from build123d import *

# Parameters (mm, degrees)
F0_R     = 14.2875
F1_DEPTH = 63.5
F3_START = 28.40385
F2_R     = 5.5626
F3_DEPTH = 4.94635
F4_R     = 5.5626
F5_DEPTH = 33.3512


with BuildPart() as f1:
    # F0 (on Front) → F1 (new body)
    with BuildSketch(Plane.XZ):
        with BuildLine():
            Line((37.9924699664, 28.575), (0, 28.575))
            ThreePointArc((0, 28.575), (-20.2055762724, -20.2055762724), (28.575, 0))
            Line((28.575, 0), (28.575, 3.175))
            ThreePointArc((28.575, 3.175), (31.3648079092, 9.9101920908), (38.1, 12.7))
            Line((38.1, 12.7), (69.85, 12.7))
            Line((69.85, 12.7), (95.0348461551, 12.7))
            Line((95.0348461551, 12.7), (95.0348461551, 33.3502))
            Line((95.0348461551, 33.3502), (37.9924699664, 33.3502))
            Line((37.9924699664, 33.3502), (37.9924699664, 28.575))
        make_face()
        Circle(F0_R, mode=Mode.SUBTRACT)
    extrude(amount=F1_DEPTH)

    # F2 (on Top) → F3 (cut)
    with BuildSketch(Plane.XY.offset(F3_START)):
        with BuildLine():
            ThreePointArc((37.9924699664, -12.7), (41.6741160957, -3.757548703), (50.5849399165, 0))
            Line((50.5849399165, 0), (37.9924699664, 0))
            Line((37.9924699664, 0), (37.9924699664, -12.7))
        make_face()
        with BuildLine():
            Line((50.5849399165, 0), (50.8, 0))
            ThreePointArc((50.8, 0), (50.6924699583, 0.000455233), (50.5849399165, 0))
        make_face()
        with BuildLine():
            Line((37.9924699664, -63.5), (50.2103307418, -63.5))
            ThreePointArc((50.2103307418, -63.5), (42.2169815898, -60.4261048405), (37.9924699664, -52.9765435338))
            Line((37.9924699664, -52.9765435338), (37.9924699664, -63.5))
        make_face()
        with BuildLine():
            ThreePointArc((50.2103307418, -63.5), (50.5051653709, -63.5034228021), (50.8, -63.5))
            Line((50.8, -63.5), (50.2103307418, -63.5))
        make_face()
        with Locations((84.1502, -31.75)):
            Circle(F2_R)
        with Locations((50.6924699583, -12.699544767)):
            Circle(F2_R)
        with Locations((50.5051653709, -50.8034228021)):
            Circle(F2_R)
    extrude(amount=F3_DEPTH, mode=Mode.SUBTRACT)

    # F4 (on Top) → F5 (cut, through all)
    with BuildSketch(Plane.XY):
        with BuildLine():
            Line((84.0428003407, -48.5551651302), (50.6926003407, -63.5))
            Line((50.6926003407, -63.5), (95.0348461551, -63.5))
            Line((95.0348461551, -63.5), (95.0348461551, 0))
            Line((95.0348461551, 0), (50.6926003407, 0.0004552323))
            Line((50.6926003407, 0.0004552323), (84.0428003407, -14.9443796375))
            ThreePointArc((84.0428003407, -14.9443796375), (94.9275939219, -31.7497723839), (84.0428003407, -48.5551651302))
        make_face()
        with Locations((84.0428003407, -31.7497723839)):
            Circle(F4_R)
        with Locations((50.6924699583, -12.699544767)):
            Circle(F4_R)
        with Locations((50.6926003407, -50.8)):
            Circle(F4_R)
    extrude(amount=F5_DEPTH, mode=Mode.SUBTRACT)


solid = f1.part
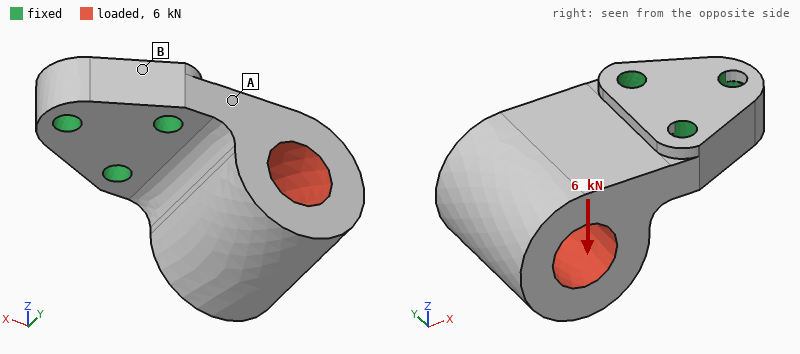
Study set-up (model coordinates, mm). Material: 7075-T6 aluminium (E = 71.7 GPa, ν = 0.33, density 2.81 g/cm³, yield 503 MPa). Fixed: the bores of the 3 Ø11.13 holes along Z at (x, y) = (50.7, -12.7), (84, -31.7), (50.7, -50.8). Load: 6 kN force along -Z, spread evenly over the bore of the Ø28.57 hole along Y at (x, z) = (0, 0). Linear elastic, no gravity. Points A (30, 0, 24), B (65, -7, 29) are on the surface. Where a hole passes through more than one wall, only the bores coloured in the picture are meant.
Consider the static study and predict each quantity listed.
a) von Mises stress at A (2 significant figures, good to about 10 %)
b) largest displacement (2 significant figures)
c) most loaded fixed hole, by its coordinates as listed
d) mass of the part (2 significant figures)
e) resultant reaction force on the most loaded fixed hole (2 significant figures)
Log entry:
30 MPa
0.22 mm
(50.7, -12.7)
540 g
3.8 kN
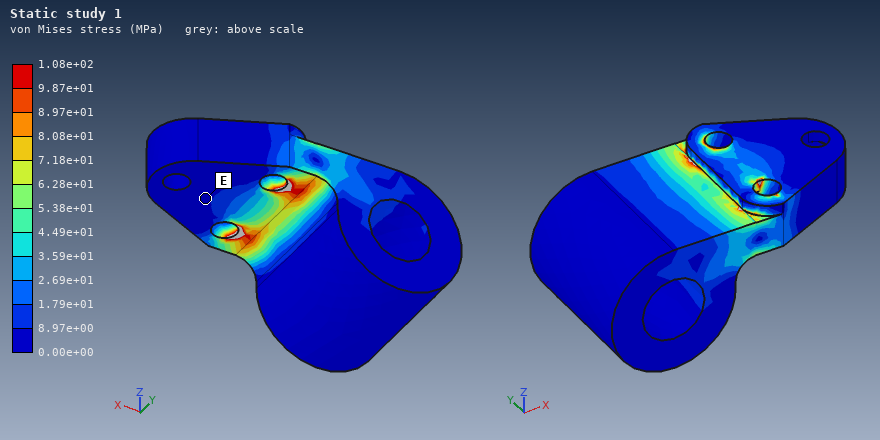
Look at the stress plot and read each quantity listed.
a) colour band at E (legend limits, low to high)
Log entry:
0.00e+00 to 8.97e+00 MPa
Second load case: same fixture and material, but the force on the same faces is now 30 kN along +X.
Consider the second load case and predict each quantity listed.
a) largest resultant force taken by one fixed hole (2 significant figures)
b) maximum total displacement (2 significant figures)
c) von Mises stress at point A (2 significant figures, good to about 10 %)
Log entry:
15 kN
0.62 mm
71 MPa
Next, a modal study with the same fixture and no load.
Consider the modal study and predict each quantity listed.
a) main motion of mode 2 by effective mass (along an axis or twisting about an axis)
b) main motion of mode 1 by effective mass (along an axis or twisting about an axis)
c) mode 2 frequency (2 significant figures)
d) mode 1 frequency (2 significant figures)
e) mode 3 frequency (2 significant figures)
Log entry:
along Y
along Z
3600 Hz
1500 Hz
5500 Hz
